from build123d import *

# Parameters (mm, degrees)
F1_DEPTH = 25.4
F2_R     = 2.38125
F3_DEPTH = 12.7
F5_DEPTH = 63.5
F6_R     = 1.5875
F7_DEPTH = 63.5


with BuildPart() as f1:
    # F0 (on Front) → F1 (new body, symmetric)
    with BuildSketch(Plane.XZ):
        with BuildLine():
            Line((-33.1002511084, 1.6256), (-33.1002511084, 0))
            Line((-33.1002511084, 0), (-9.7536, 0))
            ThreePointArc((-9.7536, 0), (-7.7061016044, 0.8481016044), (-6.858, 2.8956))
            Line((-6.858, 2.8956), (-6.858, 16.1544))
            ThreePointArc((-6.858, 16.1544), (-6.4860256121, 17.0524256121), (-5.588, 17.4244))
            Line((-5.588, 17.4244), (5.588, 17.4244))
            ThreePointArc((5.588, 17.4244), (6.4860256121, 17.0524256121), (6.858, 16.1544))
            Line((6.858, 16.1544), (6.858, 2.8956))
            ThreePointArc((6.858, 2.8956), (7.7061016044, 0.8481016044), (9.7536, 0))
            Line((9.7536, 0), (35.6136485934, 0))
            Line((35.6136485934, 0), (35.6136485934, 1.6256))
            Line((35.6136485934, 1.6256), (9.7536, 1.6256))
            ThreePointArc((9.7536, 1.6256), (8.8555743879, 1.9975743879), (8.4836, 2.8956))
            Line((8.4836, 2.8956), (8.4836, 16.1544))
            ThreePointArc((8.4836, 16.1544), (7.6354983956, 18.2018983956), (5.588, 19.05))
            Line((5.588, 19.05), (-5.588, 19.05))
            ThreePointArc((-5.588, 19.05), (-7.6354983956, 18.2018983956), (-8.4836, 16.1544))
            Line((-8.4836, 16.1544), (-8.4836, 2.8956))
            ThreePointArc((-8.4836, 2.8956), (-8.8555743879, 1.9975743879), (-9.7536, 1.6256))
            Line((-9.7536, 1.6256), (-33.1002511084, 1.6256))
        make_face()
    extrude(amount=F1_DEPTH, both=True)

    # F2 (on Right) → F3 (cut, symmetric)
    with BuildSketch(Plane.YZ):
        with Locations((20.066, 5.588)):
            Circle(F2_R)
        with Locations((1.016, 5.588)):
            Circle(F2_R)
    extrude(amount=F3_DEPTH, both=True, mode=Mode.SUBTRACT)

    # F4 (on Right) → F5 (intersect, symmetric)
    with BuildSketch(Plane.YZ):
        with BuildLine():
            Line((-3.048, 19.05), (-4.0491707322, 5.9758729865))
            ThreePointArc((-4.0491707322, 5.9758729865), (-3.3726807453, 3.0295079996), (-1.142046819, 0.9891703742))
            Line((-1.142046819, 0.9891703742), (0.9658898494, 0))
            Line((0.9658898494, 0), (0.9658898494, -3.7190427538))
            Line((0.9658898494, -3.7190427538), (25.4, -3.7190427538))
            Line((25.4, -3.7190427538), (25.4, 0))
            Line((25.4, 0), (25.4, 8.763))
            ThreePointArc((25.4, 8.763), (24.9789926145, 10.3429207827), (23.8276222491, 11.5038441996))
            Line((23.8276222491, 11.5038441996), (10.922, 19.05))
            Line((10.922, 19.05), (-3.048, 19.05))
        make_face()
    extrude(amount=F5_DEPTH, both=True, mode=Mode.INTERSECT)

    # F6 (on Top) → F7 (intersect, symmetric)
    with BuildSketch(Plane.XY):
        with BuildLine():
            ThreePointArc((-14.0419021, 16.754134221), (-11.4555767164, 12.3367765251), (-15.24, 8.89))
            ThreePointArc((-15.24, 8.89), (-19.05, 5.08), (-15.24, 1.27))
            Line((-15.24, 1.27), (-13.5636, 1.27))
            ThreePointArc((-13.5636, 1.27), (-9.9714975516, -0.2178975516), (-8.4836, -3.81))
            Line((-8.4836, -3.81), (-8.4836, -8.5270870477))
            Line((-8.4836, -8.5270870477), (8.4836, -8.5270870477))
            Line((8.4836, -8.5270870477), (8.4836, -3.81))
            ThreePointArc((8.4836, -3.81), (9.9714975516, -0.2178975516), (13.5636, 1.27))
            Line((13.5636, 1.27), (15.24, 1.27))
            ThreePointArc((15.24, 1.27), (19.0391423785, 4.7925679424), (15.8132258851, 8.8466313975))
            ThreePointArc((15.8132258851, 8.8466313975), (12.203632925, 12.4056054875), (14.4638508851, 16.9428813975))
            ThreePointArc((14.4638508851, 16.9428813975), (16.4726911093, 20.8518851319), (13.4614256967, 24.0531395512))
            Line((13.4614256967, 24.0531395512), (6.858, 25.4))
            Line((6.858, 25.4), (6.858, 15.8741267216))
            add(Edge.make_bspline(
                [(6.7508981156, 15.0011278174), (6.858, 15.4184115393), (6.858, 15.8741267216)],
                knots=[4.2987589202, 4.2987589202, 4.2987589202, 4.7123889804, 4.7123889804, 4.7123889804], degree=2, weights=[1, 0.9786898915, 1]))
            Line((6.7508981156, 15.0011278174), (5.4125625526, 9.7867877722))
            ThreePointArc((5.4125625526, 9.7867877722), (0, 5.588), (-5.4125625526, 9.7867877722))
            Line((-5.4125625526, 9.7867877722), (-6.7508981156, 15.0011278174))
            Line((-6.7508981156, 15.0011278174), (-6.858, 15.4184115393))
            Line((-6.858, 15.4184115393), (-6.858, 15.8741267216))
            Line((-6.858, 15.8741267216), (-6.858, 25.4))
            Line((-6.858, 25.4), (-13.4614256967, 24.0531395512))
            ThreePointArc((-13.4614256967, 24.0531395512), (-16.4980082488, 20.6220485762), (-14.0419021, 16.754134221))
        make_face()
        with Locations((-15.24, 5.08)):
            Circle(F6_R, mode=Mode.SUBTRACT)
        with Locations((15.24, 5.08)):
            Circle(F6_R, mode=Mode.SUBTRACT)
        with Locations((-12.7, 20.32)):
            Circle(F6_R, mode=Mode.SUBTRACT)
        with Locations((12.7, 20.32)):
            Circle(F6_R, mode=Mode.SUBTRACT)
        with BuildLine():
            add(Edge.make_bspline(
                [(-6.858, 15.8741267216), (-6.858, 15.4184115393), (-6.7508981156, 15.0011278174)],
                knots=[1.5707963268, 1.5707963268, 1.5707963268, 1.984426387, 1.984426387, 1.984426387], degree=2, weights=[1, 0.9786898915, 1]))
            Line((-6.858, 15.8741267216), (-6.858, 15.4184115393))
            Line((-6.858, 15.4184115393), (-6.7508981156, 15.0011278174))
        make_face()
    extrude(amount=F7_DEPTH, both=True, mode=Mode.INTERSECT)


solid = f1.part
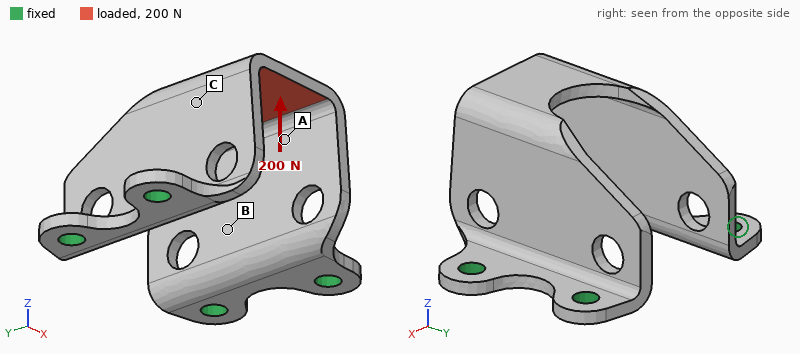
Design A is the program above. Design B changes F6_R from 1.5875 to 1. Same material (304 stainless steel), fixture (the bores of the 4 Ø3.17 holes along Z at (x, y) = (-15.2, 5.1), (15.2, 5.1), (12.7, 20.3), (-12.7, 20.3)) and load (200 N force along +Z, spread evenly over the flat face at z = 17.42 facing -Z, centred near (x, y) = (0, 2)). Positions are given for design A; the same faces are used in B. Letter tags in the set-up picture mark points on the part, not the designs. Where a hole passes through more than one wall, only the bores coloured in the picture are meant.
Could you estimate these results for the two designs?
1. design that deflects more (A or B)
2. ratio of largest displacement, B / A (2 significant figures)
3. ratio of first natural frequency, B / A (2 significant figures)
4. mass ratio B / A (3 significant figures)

B
1.2
0.99
1.01
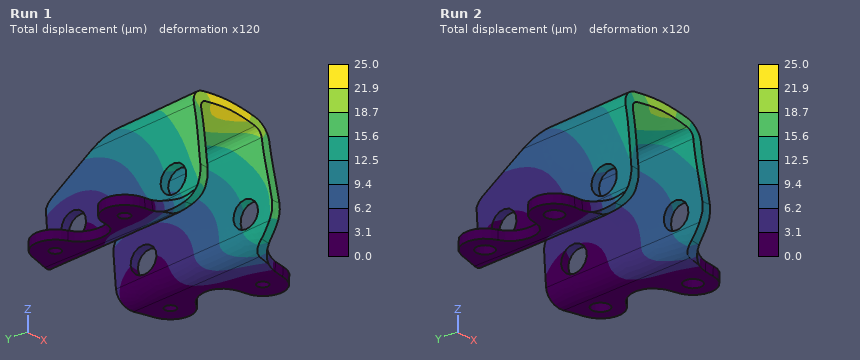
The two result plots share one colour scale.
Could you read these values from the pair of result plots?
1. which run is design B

Run 1
